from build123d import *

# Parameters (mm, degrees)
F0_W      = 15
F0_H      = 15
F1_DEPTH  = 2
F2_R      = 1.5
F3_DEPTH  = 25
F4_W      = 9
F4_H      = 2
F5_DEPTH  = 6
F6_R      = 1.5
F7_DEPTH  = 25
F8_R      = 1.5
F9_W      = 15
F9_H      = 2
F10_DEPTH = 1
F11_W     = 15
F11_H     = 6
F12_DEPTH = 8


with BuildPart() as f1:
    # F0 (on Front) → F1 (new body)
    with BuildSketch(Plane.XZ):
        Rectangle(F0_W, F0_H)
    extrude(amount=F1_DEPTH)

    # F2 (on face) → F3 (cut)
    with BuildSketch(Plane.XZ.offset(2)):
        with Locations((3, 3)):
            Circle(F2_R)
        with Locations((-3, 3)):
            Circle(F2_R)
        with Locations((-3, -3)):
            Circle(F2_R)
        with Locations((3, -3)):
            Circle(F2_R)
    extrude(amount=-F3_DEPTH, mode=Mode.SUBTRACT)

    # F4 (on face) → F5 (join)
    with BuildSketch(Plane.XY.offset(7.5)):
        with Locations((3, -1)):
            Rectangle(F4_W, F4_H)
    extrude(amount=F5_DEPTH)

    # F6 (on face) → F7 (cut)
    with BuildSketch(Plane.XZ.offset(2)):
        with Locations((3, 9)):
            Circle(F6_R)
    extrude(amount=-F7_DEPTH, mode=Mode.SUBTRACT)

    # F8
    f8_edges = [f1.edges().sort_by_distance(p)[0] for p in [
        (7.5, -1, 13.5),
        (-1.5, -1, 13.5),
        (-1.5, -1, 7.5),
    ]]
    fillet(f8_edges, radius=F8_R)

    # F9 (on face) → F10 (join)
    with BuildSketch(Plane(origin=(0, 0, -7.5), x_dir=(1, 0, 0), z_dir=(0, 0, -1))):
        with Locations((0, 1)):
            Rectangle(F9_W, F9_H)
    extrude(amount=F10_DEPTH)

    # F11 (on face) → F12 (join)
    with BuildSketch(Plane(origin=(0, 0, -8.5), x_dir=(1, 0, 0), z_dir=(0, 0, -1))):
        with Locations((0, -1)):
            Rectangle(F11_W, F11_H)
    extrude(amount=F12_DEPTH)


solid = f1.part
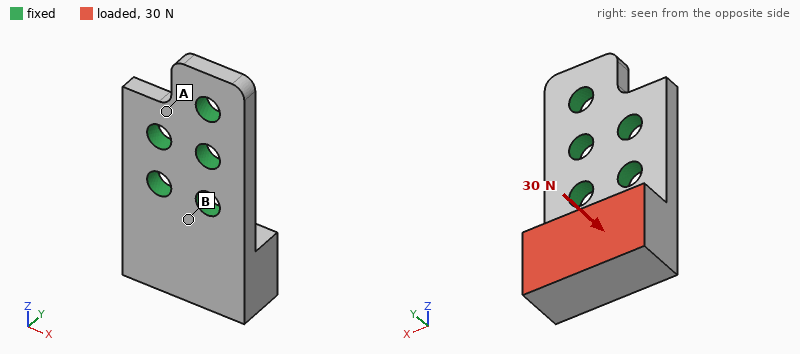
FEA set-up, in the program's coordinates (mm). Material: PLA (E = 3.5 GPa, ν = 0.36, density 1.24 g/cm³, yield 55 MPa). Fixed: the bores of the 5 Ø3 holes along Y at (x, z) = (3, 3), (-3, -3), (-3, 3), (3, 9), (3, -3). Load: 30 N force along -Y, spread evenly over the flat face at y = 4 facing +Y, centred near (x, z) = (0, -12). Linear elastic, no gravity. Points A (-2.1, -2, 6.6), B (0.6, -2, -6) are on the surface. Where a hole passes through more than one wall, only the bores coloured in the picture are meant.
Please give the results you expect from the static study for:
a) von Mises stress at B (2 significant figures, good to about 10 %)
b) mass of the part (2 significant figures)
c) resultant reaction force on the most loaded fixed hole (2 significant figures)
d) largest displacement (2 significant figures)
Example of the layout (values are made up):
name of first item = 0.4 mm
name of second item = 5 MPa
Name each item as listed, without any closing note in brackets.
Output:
von Mises stress at B = 17 MPa
mass of the part = 1.5 g
resultant reaction force on the most loaded fixed hole = 17 N
largest displacement = 0.30 mm
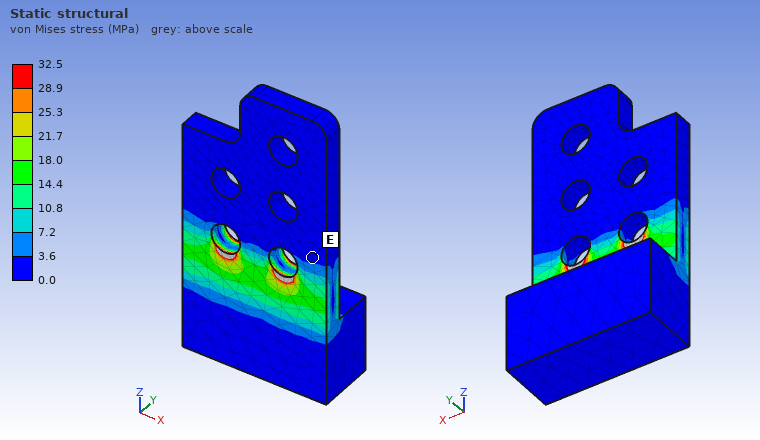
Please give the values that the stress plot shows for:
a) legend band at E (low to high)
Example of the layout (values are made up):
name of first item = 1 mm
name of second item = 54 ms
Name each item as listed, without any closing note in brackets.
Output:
legend band at E = 0.0 to 3.6 MPa
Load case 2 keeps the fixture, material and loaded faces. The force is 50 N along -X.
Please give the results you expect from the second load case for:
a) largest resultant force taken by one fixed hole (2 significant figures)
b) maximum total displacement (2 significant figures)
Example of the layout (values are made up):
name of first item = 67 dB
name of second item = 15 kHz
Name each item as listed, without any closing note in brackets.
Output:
largest resultant force taken by one fixed hole = 56 N
maximum total displacement = 94 µm
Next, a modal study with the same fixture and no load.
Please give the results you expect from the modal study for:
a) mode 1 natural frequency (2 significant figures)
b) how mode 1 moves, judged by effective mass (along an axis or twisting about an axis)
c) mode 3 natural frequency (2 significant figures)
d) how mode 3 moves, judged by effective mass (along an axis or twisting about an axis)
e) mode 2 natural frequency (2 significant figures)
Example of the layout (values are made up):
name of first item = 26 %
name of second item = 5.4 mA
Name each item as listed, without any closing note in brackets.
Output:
mode 1 natural frequency = 2000 Hz
how mode 1 moves, judged by effective mass = along Y
mode 3 natural frequency = 8200 Hz
how mode 3 moves, judged by effective mass = along X
mode 2 natural frequency = 5400 Hz
